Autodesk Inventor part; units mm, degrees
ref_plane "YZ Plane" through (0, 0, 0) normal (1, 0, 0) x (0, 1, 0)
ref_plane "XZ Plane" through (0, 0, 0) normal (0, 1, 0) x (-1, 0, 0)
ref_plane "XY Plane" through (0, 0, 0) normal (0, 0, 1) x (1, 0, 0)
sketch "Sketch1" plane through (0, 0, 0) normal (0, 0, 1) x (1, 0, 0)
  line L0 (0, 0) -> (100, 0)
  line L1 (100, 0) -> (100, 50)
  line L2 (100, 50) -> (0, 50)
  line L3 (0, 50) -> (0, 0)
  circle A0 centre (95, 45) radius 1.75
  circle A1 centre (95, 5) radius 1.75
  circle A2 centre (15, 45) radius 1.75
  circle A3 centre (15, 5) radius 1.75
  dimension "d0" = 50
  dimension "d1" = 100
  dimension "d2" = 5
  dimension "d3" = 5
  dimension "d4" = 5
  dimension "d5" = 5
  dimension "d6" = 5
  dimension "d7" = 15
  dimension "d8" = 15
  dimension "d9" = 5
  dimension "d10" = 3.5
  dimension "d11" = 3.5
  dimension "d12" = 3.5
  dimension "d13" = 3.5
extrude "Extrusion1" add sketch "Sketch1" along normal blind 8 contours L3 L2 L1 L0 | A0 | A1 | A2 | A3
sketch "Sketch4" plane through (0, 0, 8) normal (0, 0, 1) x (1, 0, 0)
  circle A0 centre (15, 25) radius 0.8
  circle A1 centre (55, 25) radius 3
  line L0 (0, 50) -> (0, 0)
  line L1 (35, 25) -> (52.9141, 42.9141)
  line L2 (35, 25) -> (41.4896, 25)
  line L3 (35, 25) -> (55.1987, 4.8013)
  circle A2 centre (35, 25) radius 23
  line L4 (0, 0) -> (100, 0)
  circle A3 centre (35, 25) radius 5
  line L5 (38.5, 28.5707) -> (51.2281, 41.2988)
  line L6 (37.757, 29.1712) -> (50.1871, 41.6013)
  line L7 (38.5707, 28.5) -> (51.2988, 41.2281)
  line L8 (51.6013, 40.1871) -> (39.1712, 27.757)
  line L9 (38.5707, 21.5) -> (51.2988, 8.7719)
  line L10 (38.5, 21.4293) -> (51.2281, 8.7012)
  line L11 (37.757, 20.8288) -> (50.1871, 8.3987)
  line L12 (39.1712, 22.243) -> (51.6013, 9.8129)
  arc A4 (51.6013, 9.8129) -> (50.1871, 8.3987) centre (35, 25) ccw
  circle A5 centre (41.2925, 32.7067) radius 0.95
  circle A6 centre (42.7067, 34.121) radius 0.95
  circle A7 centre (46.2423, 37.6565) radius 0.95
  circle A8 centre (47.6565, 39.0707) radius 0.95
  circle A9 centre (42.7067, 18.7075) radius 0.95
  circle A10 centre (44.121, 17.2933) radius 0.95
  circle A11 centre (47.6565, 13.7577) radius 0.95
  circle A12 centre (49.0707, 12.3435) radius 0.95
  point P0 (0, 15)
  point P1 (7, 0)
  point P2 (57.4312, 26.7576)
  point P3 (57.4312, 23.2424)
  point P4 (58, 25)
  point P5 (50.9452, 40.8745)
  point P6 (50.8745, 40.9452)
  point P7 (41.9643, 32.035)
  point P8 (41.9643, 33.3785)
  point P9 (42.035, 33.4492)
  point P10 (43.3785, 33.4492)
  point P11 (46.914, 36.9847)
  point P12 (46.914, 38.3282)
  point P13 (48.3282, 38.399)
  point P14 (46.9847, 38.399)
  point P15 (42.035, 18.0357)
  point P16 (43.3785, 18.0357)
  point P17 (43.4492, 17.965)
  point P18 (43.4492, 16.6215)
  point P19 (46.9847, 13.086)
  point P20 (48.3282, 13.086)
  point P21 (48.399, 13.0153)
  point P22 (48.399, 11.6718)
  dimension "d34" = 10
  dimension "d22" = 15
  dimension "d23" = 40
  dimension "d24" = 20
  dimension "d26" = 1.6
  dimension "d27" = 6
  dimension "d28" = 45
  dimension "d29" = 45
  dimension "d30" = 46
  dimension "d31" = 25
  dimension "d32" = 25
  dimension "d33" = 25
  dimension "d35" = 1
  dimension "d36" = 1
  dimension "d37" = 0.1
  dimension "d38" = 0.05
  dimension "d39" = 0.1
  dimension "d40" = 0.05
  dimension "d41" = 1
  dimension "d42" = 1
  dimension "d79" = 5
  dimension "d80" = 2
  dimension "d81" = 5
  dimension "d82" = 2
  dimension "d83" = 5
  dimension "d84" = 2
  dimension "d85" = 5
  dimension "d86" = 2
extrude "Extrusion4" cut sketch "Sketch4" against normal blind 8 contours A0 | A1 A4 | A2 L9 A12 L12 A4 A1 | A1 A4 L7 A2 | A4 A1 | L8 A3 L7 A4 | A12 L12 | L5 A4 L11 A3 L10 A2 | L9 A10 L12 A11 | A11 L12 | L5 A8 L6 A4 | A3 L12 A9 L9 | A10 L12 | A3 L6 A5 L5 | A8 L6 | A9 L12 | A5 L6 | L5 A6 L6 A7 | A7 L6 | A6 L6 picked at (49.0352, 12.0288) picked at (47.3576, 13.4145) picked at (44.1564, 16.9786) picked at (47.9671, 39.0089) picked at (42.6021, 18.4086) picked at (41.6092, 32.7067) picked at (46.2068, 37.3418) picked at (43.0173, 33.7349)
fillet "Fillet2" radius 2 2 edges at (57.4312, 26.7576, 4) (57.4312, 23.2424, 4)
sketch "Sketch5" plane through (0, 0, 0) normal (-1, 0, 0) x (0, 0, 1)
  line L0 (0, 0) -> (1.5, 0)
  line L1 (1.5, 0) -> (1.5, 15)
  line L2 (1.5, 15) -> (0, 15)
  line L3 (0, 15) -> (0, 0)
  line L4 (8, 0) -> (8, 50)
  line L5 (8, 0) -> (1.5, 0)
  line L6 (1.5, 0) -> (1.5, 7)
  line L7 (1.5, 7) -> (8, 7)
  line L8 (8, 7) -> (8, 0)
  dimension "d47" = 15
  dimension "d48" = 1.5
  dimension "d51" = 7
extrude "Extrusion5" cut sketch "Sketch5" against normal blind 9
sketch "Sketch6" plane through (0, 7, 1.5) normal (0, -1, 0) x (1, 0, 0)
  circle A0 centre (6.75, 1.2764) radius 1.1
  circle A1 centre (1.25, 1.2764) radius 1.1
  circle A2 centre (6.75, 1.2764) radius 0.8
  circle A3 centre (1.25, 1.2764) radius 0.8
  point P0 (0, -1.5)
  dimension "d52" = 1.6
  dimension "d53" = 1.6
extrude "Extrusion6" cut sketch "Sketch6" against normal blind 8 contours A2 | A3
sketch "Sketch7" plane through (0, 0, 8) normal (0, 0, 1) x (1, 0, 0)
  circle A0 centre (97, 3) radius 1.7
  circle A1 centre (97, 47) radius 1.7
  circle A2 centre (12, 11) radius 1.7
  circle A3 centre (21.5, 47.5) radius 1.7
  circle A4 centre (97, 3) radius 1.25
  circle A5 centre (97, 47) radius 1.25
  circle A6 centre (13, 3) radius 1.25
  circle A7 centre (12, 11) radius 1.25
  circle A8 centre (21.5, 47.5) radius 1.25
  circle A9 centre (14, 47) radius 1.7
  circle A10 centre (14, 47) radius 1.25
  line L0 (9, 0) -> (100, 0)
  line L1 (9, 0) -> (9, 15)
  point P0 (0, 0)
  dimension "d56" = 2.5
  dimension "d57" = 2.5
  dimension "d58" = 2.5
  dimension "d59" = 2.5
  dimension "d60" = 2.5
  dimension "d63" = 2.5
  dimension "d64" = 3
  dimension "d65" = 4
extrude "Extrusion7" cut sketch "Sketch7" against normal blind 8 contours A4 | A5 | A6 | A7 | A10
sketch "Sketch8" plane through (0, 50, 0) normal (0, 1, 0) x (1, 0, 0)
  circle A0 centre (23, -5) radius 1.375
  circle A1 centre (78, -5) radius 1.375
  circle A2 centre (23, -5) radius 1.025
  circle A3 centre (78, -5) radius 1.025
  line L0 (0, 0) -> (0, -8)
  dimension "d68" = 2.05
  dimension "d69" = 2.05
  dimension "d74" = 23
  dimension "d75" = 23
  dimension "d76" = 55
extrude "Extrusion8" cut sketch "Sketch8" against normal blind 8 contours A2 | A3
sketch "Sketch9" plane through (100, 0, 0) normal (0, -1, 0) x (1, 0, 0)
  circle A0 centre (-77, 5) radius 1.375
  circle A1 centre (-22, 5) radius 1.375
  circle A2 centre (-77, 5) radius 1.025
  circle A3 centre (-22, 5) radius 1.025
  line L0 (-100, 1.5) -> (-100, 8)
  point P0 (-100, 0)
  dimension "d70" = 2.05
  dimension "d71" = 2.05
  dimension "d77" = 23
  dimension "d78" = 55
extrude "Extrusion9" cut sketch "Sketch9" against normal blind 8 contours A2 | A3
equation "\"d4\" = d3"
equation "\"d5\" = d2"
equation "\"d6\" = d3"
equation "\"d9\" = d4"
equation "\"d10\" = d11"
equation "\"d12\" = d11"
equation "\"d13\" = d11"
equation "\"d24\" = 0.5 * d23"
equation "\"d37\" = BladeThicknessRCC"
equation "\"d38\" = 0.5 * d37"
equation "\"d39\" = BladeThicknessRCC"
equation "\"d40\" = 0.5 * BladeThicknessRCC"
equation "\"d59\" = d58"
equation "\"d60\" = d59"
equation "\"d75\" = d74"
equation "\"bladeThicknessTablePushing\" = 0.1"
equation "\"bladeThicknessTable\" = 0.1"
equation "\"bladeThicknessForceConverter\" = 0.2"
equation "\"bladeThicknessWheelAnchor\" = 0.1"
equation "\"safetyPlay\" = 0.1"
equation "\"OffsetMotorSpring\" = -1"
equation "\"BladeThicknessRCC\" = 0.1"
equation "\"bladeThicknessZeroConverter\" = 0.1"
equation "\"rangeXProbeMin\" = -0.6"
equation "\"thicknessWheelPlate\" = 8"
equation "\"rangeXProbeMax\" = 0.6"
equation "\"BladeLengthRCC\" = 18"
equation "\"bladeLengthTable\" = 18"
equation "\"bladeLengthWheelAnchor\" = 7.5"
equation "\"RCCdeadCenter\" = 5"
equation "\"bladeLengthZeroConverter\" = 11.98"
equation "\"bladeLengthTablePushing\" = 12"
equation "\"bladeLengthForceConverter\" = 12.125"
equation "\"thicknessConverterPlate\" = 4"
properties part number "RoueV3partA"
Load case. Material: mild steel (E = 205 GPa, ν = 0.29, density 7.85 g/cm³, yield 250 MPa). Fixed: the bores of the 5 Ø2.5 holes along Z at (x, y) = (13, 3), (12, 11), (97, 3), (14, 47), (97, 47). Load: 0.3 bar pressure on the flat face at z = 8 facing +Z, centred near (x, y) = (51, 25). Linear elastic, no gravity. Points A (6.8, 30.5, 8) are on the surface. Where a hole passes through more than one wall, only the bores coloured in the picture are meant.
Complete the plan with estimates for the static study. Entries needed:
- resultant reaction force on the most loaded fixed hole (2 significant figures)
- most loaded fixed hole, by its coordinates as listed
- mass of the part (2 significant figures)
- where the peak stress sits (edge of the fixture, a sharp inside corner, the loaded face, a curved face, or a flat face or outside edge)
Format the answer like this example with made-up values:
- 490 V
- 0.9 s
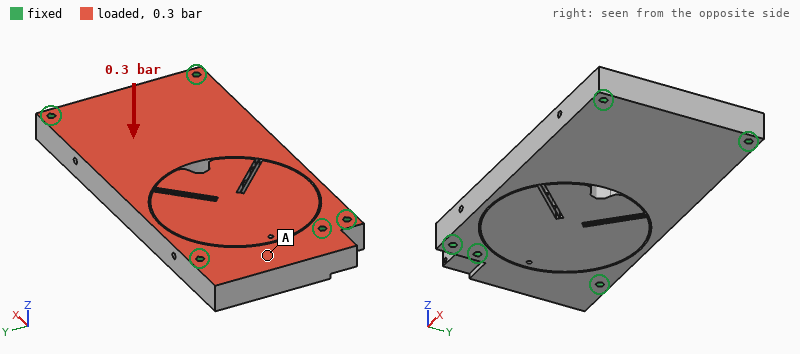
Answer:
- 38 N
- (14, 47)
- 300 g
- a flat face or outside edge
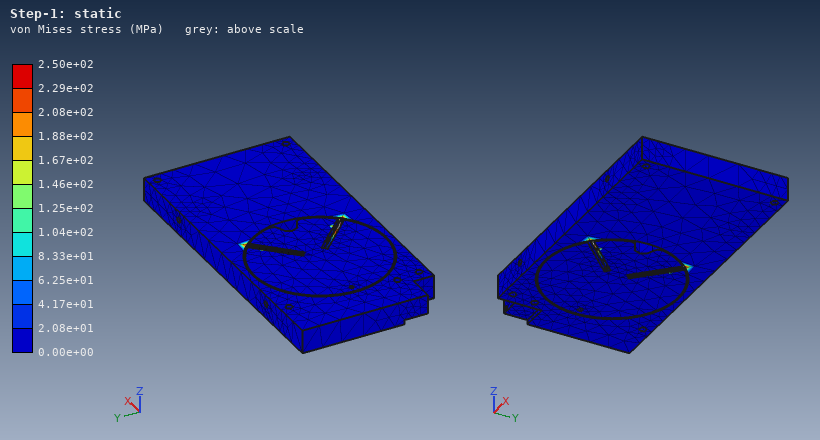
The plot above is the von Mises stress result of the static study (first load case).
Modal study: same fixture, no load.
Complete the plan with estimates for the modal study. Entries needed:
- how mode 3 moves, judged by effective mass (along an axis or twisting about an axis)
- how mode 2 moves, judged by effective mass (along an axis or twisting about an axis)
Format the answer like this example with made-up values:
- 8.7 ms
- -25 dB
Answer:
- along Y
- along Z
